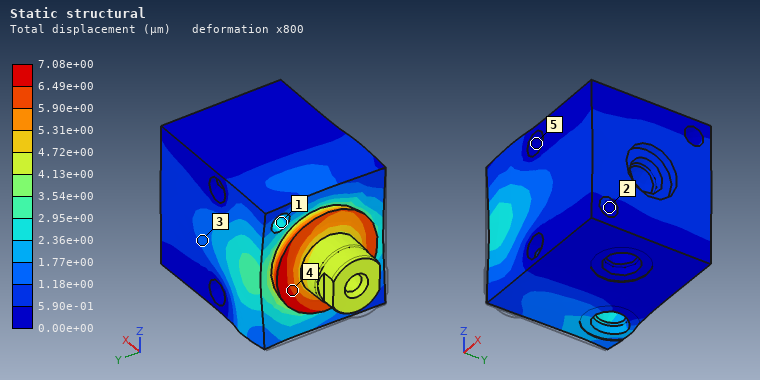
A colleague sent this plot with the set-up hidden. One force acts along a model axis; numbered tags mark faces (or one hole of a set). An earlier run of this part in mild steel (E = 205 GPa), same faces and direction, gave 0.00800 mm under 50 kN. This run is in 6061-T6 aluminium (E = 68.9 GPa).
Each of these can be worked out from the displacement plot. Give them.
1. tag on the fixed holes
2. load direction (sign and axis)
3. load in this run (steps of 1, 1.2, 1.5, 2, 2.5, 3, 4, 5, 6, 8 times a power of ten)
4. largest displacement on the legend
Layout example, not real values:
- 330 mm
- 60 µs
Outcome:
- 5
- +X
- 15 kN
- 7.08e+00 µm
